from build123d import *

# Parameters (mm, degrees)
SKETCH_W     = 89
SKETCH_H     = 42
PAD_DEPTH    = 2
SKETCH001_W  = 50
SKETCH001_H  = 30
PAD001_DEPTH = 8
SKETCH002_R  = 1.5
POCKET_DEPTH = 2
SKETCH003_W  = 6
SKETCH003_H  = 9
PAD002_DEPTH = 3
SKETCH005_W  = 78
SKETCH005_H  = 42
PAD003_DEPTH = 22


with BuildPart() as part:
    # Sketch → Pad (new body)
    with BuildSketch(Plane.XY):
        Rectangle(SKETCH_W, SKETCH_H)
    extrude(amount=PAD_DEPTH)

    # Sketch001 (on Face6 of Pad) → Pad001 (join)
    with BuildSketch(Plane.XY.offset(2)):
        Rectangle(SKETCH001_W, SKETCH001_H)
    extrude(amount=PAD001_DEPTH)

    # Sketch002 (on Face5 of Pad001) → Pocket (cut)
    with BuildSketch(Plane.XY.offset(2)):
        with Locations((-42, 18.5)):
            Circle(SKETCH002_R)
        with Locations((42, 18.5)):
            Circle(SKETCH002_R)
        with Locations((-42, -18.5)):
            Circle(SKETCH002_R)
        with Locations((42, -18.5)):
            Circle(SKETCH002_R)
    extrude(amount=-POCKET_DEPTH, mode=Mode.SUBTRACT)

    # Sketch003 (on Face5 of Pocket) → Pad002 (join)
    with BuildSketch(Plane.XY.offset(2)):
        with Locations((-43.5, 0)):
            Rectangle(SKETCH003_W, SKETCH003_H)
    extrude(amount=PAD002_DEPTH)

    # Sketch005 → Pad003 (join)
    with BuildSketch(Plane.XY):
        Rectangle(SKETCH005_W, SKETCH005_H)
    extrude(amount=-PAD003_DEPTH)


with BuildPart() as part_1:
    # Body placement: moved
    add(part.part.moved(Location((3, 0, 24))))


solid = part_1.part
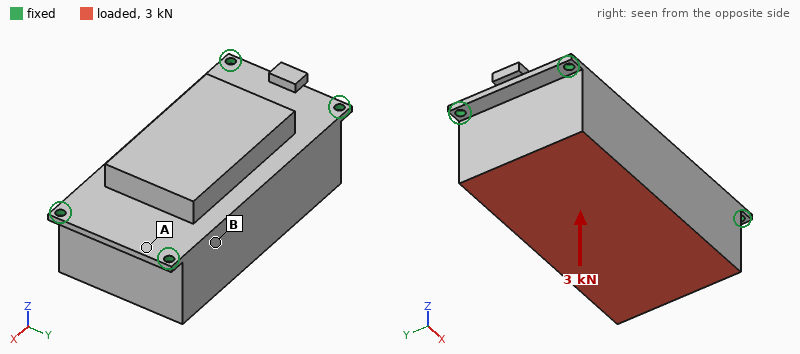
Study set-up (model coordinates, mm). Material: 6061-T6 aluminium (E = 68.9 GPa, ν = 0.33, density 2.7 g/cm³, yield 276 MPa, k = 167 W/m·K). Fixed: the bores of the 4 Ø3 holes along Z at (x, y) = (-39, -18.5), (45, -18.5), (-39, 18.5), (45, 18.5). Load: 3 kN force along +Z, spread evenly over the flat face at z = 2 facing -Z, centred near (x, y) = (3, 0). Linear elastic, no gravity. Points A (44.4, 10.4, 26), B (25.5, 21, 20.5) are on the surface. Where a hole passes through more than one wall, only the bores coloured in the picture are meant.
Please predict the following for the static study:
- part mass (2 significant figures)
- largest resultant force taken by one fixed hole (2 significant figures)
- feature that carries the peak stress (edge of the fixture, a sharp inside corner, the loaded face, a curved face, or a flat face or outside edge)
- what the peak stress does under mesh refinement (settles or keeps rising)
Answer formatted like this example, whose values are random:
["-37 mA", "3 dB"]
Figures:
["250 g", "870 N", "edge of the fixture", "keeps rising"]
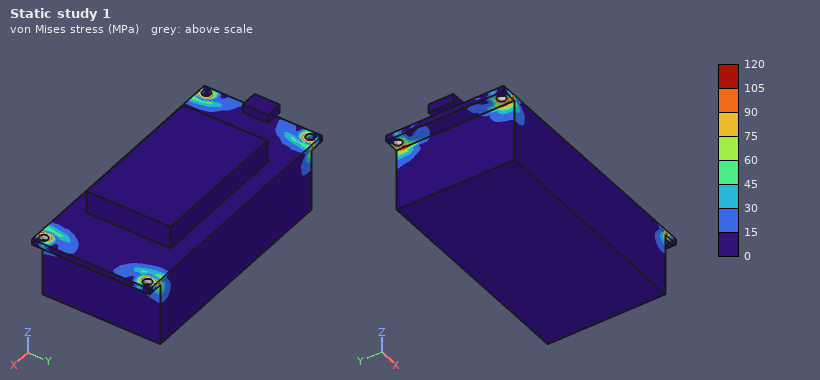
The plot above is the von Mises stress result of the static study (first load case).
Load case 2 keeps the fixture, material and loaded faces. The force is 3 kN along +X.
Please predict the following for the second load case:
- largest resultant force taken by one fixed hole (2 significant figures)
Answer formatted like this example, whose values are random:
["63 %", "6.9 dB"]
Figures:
["890 N"]
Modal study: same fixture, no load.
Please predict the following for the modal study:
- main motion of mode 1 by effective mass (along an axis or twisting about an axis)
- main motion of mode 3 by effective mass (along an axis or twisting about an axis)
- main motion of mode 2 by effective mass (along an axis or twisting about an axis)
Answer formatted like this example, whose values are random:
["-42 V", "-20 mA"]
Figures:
["along Z", "along X", "along Y"]
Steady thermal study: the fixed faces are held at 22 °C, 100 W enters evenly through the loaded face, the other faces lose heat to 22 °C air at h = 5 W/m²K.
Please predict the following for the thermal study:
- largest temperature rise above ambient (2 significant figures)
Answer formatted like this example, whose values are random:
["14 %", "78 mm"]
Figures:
["48 K"]
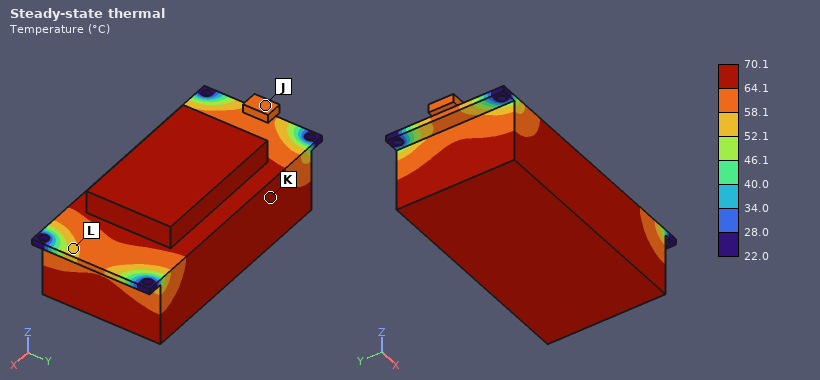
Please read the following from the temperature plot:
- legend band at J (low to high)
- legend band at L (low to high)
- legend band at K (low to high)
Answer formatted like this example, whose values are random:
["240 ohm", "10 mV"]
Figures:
["58.1 to 64.1 °C", "52.1 to 58.1 °C", "64.1 to 70.1 °C"]
